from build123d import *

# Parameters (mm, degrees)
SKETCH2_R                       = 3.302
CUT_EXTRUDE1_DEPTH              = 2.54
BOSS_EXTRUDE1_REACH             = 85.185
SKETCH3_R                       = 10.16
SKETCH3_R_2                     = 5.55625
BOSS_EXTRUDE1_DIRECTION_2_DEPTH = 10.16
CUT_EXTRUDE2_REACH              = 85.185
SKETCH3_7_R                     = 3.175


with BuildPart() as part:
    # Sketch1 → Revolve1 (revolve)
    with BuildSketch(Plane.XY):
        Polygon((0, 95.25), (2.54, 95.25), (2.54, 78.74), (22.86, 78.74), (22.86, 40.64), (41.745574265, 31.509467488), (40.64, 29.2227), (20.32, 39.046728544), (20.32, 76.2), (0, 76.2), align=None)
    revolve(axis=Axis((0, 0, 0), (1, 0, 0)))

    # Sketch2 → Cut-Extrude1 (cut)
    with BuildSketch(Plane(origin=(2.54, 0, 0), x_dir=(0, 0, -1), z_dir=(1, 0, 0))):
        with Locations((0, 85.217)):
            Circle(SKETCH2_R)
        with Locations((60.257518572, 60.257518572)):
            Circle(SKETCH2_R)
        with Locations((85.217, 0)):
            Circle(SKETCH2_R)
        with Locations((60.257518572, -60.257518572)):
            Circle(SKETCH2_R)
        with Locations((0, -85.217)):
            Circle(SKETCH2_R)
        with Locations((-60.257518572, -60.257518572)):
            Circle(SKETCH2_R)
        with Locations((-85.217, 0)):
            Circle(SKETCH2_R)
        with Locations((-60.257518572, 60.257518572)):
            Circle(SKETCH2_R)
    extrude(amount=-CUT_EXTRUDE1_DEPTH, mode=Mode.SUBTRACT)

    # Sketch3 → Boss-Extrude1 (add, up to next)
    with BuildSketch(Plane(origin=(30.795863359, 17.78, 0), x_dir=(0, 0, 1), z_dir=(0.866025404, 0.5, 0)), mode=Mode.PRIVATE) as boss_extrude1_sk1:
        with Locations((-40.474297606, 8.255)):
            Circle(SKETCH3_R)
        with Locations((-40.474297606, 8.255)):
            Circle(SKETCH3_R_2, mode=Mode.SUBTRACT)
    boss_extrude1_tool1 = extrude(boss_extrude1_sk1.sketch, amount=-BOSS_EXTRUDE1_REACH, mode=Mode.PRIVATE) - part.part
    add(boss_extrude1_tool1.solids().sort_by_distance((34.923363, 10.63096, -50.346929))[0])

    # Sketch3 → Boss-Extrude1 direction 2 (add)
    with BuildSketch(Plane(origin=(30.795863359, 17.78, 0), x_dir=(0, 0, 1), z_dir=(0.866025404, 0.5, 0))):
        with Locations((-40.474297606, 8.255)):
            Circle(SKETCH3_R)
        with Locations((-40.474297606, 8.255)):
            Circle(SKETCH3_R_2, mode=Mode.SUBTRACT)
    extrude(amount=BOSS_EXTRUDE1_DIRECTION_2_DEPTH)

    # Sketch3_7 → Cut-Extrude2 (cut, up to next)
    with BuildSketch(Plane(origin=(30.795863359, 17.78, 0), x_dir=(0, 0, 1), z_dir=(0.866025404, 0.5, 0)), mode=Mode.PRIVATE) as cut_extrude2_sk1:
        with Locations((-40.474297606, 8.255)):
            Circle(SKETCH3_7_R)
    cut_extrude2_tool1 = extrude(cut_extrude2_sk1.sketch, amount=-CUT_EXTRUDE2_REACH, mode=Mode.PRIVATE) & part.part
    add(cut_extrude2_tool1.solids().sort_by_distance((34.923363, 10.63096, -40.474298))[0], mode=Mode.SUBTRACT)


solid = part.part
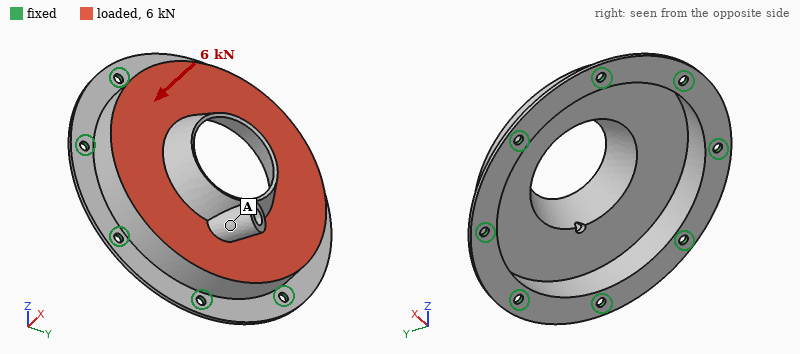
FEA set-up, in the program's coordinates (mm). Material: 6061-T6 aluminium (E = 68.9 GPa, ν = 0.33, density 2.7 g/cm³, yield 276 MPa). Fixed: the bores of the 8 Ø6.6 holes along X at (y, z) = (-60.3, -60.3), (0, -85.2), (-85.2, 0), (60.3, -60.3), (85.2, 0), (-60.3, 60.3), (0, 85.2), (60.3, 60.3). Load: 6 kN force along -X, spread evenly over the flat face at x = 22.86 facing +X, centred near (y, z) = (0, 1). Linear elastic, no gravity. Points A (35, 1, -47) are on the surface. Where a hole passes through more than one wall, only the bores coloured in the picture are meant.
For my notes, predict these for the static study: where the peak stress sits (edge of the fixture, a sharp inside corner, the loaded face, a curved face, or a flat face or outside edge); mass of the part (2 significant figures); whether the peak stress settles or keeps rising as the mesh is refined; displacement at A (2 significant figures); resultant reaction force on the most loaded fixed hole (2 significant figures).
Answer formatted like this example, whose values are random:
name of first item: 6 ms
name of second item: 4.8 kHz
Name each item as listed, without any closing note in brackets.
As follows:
where the peak stress sits: edge of the fixture
mass of the part: 270 g
whether the peak stress settles or keeps rising as the mesh is refined: keeps rising
displacement at A: 0.29 mm
resultant reaction force on the most loaded fixed hole: 870 N
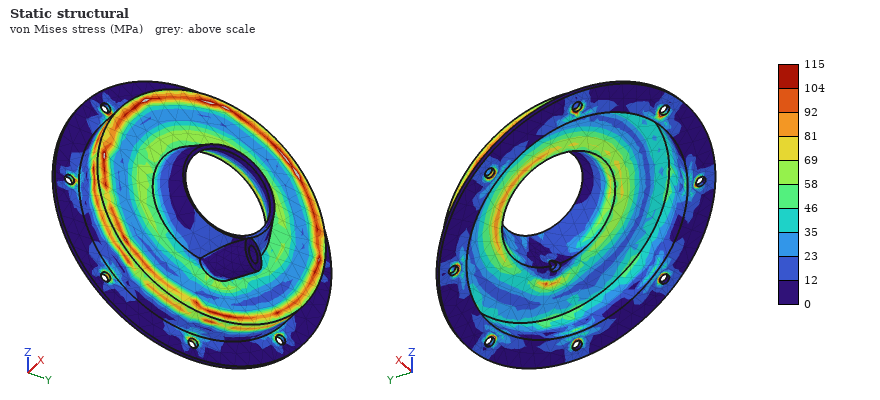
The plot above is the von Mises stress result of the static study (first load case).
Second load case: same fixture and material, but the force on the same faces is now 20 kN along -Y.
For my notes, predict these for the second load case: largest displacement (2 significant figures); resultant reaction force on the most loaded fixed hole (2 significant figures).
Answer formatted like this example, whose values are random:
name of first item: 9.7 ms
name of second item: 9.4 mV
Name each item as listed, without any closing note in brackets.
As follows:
largest displacement: 0.13 mm
resultant reaction force on the most loaded fixed hole: 4.1 kN
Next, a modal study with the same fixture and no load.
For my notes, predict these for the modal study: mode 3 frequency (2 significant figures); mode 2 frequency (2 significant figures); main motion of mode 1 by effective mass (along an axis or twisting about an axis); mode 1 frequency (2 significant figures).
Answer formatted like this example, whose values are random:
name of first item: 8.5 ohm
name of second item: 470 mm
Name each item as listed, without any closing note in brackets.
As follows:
mode 3 frequency: 2200 Hz
mode 2 frequency: 2100 Hz
main motion of mode 1 by effective mass: along X
mode 1 frequency: 1500 Hz
